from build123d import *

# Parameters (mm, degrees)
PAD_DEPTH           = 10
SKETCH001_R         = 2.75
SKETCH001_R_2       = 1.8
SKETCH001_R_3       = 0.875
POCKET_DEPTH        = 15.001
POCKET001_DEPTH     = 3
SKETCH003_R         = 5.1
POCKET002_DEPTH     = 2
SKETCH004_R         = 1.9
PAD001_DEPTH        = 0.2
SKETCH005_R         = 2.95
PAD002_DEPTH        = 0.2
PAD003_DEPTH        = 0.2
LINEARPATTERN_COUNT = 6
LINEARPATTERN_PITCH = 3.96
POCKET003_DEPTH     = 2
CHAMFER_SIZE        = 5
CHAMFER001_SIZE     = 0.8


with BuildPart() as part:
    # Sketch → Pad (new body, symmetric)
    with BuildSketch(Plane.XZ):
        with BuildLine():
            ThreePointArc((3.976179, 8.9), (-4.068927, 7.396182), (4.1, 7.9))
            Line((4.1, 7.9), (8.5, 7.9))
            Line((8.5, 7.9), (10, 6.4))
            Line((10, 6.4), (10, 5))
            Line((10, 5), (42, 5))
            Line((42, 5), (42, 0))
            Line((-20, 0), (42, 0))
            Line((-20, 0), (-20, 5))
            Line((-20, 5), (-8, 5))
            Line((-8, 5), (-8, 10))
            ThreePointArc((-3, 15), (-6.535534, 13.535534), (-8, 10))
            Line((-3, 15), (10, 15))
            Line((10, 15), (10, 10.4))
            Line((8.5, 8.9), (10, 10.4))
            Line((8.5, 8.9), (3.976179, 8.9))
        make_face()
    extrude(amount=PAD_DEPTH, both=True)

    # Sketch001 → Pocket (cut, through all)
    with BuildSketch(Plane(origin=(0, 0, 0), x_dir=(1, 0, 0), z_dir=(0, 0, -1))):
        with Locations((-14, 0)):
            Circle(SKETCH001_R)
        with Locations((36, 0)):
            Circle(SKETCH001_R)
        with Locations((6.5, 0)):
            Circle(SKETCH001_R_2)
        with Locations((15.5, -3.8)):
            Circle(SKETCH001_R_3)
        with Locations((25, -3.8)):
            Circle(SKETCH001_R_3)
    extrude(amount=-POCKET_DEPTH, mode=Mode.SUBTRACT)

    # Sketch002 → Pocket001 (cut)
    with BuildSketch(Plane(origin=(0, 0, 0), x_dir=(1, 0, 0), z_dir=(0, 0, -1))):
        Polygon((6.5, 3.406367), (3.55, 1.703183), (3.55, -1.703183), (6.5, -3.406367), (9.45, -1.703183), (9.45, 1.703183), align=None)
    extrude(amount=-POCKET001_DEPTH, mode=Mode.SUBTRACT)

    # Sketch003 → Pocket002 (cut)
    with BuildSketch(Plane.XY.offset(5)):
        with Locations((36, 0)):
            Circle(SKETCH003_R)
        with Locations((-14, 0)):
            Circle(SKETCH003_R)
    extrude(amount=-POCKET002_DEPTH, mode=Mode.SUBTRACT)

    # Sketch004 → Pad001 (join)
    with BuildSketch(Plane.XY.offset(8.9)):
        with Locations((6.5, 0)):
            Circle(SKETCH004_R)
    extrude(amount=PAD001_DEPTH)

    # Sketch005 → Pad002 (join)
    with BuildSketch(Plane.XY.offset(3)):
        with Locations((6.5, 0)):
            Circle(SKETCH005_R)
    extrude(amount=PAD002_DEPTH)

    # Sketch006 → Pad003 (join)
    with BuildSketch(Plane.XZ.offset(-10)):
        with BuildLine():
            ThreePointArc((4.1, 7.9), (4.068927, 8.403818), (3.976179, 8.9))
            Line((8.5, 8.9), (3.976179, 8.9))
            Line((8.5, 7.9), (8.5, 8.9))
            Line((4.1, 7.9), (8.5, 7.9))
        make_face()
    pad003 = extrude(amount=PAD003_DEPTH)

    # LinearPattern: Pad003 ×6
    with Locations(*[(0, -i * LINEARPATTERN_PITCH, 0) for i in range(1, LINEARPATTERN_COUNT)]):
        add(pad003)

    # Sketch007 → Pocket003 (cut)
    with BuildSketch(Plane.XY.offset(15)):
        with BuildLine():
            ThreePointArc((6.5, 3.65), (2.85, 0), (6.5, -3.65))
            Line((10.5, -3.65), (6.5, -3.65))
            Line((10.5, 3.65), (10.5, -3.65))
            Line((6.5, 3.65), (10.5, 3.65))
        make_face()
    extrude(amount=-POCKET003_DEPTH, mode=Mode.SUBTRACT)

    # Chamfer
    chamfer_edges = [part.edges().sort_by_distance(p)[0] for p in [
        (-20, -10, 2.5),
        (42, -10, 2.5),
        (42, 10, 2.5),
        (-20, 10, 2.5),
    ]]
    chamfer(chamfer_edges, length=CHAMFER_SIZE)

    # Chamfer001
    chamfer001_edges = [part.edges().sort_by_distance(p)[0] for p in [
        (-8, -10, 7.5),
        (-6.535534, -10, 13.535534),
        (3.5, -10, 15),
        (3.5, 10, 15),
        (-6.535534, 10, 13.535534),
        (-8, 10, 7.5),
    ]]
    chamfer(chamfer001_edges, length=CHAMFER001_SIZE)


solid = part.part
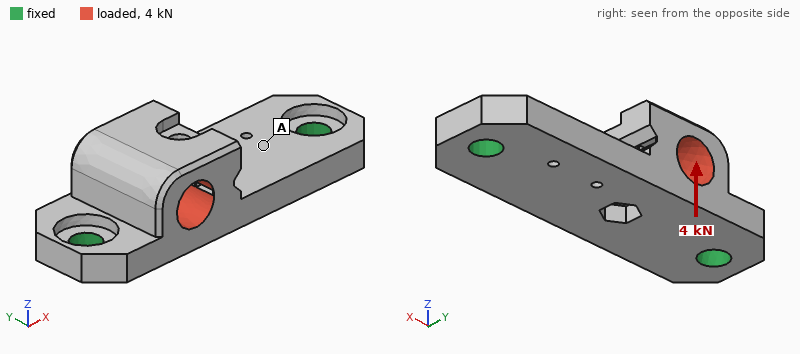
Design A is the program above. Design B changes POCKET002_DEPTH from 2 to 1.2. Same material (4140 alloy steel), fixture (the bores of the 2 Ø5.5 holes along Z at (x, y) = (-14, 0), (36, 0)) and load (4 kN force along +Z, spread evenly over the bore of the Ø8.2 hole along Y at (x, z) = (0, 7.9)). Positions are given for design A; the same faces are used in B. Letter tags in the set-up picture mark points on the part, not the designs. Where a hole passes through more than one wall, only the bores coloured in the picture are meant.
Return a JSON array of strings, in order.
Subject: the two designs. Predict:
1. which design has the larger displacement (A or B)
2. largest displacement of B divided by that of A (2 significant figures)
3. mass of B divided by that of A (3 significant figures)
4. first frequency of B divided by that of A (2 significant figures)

["A", "0.89", "1.01", "1.1"]
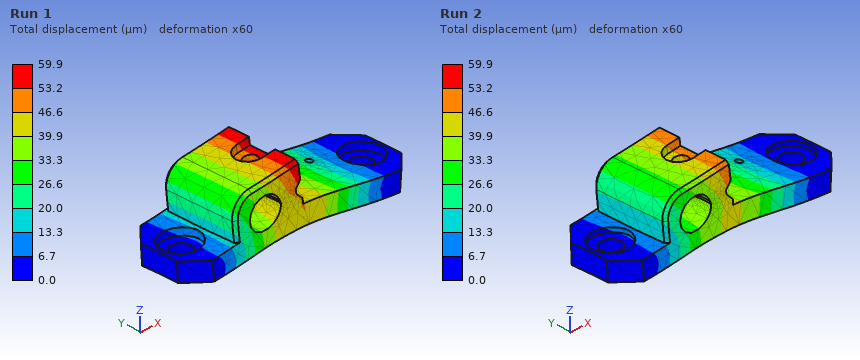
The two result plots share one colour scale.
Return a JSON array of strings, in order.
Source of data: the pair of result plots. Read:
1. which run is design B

["Run 2"]
